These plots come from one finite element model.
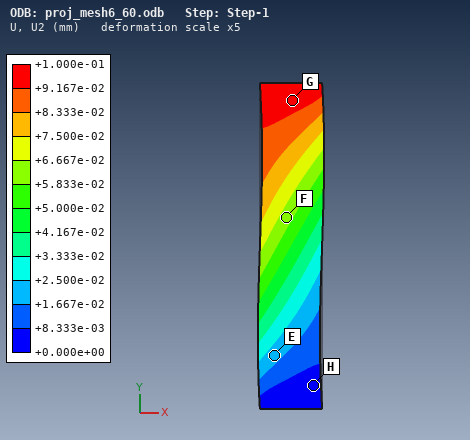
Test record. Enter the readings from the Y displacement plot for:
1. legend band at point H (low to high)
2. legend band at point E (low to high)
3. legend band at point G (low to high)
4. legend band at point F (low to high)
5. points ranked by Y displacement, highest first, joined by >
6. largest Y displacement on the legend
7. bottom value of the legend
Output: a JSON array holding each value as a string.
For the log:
["+0.000e+00 to +8.333e-03 mm", "+1.667e-02 to +2.500e-02 mm", "+9.167e-02 to +1.000e-01 mm", "+5.833e-02 to +6.667e-02 mm", "G > F > E > H", "+1.000e-01 mm", "+0.000e+00 mm"]
